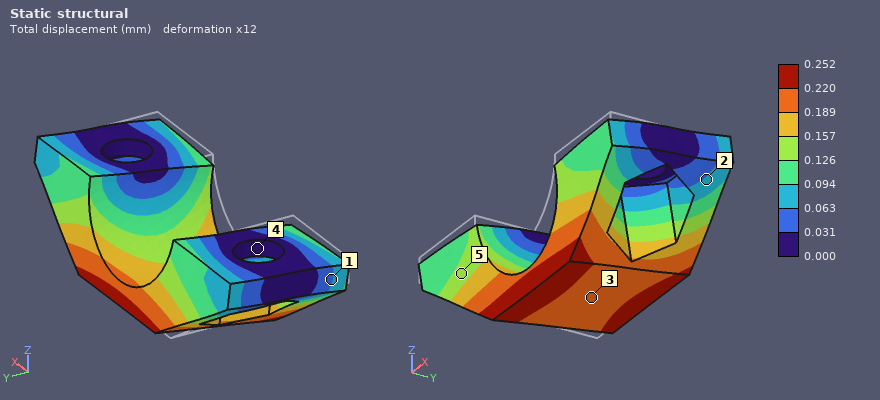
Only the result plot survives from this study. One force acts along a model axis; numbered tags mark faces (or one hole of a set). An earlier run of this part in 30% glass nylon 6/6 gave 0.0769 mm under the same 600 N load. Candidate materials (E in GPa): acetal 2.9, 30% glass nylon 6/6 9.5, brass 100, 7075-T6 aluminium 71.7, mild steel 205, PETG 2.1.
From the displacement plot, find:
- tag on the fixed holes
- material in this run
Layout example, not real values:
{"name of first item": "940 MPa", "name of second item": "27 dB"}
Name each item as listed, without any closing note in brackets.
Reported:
{"tag on the fixed holes": "4", "material in this run": "acetal"}
